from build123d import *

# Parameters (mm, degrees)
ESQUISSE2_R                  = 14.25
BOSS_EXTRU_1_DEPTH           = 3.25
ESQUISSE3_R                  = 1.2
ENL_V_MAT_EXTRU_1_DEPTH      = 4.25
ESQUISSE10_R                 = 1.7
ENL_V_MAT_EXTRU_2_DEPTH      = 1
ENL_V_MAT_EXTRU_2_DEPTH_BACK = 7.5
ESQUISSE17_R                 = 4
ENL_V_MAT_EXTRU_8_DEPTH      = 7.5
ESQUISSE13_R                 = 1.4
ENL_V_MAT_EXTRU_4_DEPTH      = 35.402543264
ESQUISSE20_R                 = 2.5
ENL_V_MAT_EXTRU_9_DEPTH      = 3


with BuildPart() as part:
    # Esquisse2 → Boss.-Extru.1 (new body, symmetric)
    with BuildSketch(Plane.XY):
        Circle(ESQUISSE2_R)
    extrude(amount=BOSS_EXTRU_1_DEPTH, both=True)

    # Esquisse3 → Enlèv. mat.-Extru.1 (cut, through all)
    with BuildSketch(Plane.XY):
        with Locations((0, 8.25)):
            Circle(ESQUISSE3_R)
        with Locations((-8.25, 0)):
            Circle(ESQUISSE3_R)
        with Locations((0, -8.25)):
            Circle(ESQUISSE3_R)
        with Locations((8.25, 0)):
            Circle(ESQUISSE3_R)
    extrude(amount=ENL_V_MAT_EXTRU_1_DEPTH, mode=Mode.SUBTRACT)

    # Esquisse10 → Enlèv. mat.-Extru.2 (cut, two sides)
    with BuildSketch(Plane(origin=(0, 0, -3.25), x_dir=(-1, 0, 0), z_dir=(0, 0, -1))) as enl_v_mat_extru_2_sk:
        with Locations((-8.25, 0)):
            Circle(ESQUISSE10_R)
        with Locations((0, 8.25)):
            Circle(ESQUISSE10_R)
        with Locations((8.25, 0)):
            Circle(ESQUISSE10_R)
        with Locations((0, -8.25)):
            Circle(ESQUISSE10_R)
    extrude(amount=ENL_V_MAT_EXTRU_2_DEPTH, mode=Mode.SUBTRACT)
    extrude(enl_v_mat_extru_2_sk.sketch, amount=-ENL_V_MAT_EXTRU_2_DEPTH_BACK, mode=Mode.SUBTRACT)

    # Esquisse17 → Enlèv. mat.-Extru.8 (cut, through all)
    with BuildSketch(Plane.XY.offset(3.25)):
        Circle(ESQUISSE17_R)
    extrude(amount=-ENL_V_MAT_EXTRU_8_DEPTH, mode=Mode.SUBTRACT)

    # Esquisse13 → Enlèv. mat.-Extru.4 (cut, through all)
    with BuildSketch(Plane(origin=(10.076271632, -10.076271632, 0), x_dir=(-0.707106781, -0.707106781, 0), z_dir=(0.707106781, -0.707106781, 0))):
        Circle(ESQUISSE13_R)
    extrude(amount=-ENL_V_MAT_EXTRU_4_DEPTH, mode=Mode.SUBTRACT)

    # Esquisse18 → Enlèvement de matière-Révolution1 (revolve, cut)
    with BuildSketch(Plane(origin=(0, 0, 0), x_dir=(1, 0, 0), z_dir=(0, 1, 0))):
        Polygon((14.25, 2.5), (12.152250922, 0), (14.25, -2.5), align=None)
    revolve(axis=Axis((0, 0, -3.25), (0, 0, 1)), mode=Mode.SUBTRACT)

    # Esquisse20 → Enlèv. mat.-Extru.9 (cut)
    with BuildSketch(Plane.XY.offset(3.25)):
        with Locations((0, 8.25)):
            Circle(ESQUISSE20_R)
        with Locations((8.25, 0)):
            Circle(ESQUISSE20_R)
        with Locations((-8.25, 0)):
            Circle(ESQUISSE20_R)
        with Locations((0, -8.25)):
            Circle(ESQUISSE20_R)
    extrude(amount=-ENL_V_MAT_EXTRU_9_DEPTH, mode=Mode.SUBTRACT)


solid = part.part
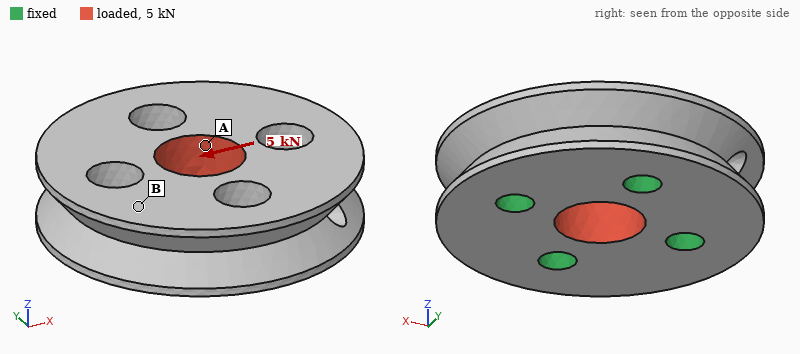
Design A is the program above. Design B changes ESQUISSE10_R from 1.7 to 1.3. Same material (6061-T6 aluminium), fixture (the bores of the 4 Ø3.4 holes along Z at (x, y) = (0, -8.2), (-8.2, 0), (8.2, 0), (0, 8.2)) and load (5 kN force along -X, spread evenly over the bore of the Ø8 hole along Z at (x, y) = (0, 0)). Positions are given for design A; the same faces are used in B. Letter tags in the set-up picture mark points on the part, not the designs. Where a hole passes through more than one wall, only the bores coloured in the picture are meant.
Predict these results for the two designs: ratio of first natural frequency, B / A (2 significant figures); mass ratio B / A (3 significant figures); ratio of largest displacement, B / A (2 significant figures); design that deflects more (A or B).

0.89
1.02
1.1
B
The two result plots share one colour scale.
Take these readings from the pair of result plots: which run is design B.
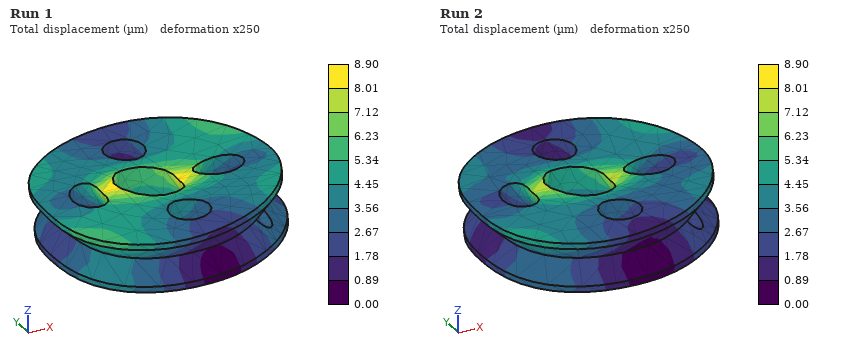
Run 1
